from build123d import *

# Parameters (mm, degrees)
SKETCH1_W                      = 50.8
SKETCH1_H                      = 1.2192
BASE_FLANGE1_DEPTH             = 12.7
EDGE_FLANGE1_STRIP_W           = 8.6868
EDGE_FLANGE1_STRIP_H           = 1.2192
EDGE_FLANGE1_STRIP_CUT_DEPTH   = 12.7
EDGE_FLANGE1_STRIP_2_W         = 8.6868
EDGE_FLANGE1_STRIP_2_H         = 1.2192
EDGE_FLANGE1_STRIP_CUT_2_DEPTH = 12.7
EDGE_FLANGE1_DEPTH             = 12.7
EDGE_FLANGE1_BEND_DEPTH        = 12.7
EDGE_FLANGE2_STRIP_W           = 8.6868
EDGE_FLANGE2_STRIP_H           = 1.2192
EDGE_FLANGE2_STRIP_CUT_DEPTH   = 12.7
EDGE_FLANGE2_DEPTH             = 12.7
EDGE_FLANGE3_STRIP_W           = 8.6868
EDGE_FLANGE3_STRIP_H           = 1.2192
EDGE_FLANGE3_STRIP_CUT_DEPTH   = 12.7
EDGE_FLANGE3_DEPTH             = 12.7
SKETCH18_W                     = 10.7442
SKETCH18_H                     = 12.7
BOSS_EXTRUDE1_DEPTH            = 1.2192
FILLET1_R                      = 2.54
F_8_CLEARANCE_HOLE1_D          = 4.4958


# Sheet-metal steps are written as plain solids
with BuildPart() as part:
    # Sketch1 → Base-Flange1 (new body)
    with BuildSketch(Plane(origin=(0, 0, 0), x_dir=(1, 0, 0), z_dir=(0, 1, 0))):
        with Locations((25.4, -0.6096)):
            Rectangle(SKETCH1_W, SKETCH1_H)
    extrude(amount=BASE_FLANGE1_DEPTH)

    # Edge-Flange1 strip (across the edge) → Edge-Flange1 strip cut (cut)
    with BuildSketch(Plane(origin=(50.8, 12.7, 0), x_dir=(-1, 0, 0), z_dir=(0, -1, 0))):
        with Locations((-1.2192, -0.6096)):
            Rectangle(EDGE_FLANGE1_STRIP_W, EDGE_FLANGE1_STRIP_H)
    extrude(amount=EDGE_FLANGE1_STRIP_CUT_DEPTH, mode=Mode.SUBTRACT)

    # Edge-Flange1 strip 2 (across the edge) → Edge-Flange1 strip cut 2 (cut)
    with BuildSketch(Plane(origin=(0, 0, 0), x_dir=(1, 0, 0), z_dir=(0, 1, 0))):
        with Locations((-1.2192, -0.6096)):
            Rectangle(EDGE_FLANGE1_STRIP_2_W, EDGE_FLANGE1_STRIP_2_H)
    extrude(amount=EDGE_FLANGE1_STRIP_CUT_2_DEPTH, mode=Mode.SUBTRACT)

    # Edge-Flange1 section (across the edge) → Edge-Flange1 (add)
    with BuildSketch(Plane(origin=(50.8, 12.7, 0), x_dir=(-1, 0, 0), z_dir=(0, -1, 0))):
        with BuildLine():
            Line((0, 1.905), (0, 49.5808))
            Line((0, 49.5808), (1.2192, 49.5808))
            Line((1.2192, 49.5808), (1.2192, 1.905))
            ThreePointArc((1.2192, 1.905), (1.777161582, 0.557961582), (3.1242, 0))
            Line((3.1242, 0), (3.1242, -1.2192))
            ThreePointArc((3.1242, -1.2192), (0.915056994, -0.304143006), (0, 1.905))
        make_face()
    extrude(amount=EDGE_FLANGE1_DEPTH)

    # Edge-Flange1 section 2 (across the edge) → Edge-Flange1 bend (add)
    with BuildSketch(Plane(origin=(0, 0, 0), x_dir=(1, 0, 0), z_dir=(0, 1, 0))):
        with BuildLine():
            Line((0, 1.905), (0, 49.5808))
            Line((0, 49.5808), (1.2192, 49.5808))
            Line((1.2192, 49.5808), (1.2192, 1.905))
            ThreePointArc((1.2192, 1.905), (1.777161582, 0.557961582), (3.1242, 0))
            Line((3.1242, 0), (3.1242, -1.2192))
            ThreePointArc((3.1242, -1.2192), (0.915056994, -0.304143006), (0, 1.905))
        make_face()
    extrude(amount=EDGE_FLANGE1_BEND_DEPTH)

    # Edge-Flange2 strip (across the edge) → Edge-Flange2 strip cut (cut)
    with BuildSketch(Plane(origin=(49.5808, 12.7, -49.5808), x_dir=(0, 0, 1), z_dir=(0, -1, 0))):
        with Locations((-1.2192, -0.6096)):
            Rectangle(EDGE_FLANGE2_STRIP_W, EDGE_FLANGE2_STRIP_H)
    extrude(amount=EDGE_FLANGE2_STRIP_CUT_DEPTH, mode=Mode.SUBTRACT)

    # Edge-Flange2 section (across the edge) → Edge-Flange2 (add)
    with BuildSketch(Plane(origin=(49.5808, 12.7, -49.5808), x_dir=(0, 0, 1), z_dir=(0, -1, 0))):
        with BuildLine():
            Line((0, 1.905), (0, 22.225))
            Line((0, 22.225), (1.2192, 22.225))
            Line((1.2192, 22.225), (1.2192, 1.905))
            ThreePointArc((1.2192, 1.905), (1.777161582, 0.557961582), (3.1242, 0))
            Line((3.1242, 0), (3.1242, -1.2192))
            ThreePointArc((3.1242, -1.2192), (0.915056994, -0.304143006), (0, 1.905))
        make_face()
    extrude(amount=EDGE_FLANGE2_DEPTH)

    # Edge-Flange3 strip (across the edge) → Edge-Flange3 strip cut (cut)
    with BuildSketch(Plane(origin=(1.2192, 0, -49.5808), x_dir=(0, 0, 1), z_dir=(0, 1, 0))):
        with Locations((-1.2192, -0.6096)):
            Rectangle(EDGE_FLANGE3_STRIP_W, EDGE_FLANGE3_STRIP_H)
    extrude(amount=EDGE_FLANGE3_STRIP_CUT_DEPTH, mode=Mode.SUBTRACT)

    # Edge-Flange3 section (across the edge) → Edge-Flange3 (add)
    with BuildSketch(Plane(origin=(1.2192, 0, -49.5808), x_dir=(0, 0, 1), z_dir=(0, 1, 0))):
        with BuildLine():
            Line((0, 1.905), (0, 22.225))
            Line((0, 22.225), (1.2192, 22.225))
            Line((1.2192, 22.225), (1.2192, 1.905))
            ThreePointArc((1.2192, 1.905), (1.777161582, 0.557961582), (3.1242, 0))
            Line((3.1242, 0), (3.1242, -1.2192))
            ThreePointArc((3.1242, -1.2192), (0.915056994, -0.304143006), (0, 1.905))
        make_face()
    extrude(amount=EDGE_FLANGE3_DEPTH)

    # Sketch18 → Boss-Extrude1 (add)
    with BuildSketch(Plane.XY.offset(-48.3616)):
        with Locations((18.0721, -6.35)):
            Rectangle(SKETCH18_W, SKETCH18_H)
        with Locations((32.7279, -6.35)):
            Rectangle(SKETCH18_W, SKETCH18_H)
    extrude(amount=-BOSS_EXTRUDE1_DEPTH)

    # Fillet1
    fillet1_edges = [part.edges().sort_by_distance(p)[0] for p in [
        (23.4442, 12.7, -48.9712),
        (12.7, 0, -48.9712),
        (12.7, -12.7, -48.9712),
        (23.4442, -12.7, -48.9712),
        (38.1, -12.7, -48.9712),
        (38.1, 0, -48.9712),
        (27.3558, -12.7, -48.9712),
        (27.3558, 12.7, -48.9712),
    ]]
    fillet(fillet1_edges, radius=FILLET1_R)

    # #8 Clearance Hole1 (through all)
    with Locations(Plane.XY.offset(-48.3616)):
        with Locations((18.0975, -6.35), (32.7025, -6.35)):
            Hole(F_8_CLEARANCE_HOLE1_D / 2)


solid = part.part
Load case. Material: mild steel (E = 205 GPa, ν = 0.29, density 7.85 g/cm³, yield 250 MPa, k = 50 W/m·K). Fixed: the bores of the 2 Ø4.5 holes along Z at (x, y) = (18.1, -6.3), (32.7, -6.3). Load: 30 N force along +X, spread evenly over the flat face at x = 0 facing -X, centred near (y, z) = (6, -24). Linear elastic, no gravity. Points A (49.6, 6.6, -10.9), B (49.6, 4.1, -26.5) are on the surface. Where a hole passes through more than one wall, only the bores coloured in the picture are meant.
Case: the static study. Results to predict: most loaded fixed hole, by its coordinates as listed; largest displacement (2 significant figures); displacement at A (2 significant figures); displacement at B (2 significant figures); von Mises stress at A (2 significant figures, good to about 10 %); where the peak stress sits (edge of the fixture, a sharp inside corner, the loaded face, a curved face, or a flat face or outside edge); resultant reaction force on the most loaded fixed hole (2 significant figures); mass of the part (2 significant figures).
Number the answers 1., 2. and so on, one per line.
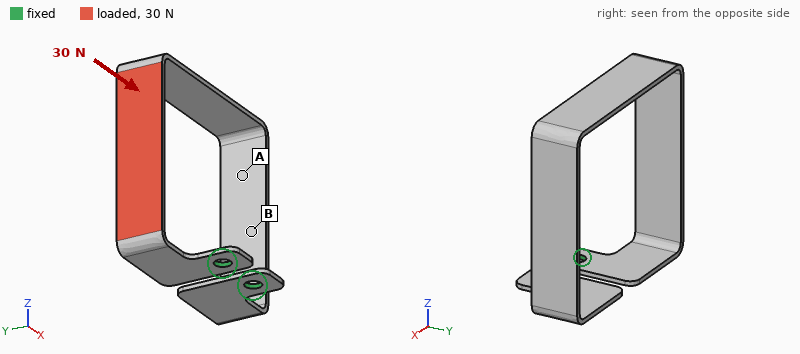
1. (18.1, -6.3)
2. 0.77 mm
3. 0.60 mm
4. 0.36 mm
5. 32 MPa
6. a flat face or outside edge
7. 23 N
8. 25 g
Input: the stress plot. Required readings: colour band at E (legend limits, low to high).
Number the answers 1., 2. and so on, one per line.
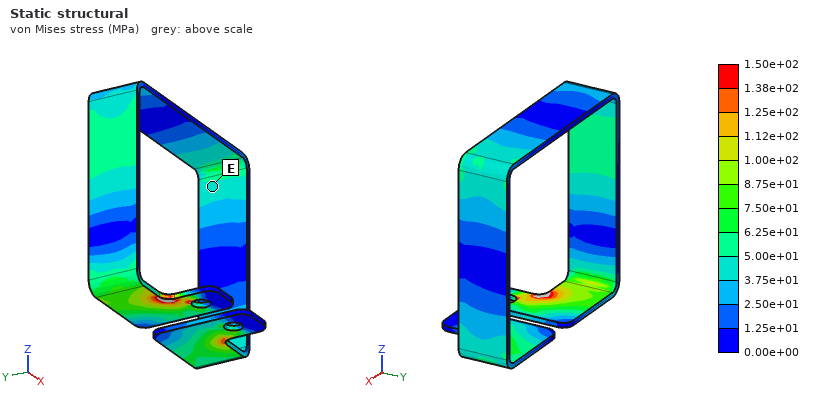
1. 3.75e+01 to 5.00e+01 MPa
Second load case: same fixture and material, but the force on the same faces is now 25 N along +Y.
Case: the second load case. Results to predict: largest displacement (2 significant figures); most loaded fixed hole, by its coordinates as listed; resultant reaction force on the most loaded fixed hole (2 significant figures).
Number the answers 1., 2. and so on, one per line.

1. 0.85 mm
2. (18.1, -6.3)
3. 22 N
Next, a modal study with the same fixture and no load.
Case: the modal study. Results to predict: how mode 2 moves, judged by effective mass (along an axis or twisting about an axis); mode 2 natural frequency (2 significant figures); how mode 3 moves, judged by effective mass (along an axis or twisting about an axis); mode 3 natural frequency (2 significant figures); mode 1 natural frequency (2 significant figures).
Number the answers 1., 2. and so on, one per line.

1. along X
2. 220 Hz
3. twisting about Z
4. 590 Hz
5. 210 Hz
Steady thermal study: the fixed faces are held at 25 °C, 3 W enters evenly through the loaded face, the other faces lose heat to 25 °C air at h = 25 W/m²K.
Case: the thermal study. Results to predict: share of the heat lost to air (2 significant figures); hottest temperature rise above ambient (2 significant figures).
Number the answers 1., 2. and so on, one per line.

1. 68 %
2. 53 K
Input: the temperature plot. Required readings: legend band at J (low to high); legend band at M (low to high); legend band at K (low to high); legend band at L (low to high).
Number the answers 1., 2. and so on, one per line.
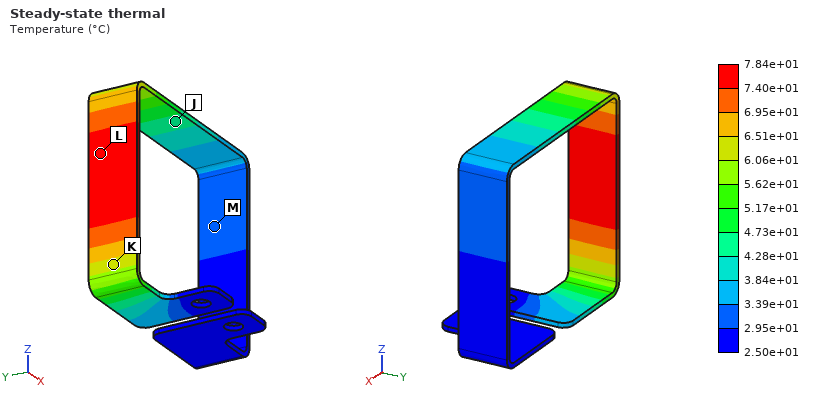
1. 4.28e+01 to 4.73e+01 °C
2. 2.95e+01 to 3.39e+01 °C
3. 6.06e+01 to 6.51e+01 °C
4. 7.40e+01 to 7.84e+01 °C
